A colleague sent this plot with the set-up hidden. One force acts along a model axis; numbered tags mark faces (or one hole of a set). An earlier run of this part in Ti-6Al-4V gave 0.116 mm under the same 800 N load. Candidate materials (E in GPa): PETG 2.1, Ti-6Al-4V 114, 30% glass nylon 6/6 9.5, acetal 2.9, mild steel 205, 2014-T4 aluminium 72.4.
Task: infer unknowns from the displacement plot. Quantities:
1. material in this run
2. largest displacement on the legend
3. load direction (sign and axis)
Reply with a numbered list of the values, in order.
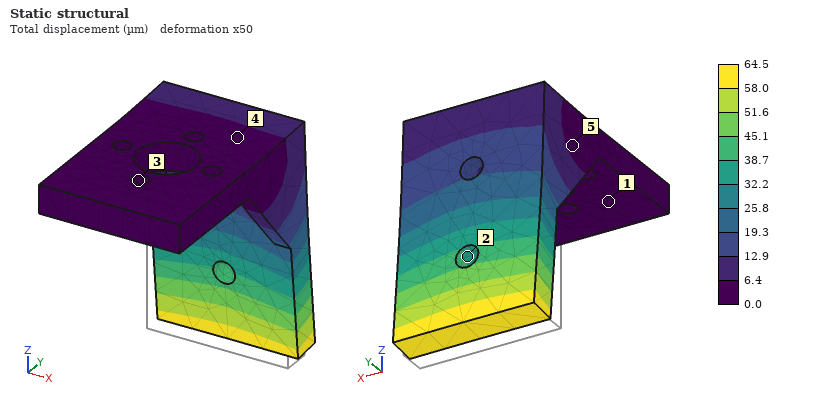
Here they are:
1. mild steel
2. 64.5 µm
3. +Y
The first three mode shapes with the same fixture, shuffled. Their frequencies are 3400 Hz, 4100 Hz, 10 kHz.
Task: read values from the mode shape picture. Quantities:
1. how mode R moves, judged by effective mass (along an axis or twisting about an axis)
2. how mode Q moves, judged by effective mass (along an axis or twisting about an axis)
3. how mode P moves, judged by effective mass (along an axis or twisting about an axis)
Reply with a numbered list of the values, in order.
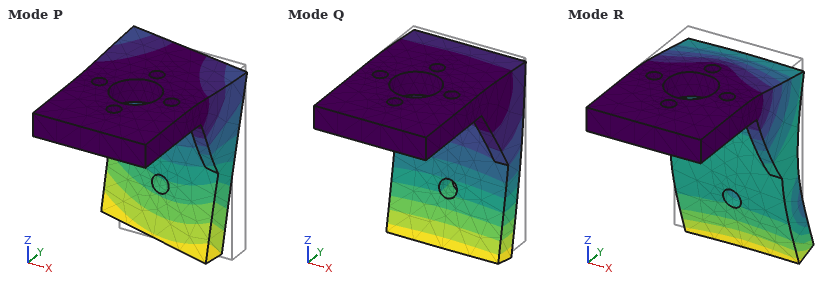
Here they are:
1. along Z
2. along Y
3. along X
